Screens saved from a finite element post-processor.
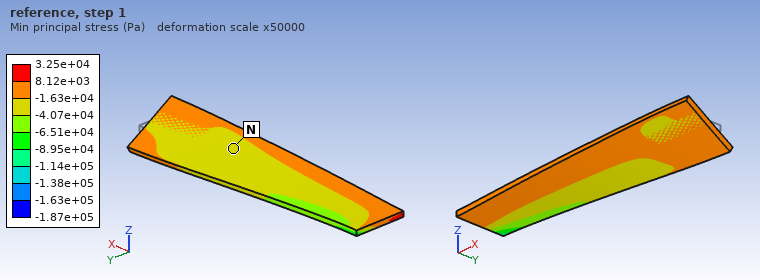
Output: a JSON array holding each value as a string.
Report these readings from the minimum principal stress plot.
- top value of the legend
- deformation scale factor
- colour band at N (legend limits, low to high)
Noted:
["3.25e+04 Pa", "50000", "-4.07e+04 to -1.63e+04 Pa"]
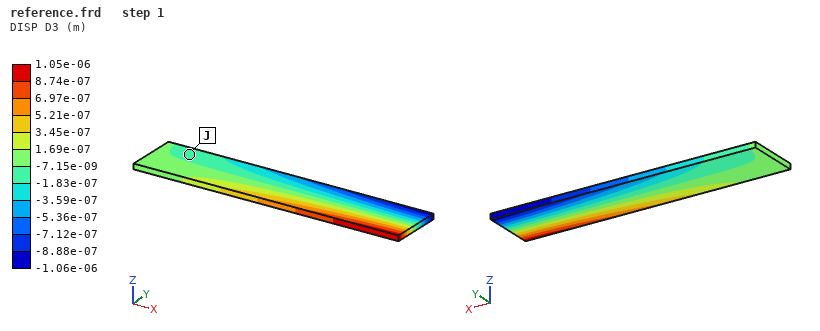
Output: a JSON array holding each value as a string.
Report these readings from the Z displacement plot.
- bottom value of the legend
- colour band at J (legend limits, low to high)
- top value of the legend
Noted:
["-1.06e-06 m", "-1.83e-07 to -7.15e-09 m", "1.05e-06 m"]
